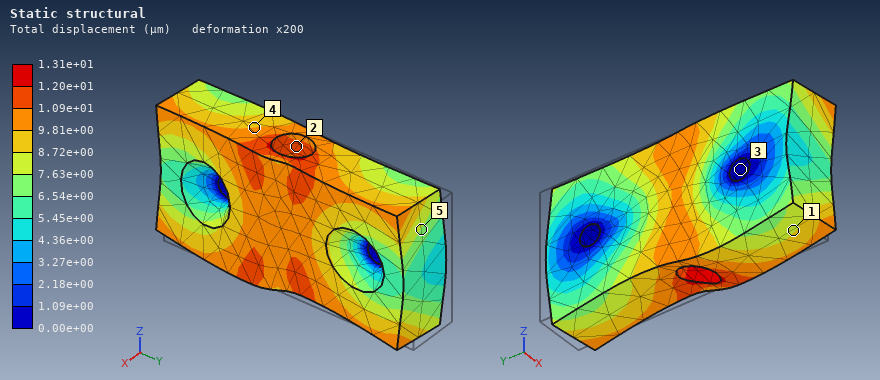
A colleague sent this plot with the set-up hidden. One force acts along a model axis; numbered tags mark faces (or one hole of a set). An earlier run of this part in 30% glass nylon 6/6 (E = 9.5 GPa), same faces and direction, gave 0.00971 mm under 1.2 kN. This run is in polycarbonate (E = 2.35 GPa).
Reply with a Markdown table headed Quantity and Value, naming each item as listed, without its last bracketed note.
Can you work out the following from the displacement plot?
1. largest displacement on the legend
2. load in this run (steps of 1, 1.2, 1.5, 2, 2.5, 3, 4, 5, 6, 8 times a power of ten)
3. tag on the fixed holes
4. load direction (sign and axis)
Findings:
| Quantity | Value |
|---|---|
| largest displacement on the legend | 1.31e+01 µm |
| load in this run | 400 N |
| tag on the fixed holes | 3 |
| load direction | -Y |
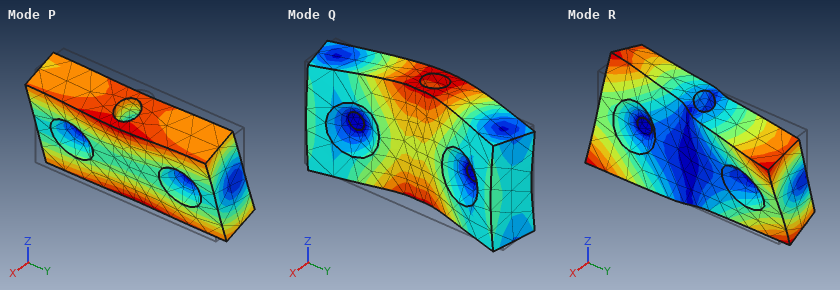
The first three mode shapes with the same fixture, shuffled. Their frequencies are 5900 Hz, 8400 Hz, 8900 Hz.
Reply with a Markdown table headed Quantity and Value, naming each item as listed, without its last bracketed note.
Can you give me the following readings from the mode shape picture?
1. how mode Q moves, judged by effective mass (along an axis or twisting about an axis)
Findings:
| Quantity | Value |
|---|---|
| how mode Q moves, judged by effective mass | along X |
